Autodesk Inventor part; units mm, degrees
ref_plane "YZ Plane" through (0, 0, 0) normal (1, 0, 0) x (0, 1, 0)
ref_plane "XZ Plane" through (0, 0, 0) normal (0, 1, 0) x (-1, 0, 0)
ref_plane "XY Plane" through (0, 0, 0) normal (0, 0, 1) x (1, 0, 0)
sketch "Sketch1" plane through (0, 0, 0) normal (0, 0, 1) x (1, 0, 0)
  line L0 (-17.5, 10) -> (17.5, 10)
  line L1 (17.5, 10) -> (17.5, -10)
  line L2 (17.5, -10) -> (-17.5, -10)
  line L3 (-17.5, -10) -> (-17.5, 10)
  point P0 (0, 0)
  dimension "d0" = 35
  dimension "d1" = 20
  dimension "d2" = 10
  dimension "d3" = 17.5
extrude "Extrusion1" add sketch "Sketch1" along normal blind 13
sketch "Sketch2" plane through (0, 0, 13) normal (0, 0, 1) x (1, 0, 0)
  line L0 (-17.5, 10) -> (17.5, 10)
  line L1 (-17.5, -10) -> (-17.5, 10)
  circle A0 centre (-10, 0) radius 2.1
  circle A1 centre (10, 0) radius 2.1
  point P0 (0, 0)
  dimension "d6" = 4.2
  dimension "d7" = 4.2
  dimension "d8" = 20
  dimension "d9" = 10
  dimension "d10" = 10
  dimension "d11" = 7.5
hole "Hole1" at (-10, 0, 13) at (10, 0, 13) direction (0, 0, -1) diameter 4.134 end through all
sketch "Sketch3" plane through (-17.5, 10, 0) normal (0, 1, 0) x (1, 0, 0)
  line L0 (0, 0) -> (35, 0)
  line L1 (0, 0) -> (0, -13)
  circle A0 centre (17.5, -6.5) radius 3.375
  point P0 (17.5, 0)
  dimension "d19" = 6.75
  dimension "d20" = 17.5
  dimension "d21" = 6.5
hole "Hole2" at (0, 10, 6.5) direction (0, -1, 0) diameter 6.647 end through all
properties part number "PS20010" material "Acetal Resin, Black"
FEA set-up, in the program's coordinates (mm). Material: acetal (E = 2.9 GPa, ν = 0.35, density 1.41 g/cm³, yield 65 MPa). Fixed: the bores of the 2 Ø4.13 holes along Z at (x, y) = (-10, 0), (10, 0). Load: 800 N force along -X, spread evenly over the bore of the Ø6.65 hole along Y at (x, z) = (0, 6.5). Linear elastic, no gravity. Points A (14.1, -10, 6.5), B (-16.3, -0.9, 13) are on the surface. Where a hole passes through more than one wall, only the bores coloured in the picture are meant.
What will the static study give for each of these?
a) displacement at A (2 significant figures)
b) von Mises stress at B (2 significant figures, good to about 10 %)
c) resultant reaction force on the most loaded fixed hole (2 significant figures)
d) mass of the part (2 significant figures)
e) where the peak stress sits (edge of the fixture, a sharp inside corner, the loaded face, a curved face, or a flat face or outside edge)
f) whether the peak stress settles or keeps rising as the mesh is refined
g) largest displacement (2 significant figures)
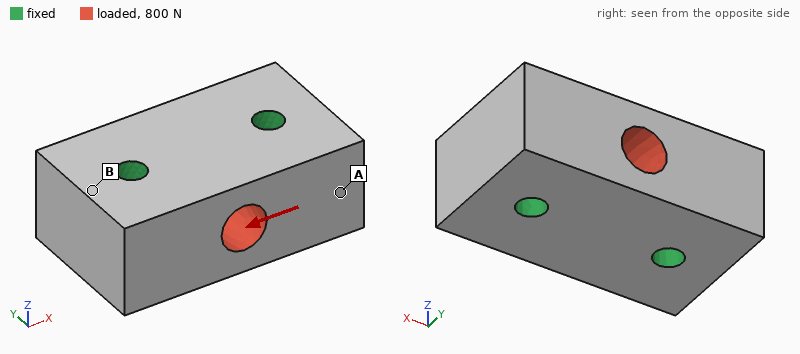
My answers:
5.5 µm
0.98 MPa
400 N
11 g
edge of the fixture
keeps rising
9.6 µm
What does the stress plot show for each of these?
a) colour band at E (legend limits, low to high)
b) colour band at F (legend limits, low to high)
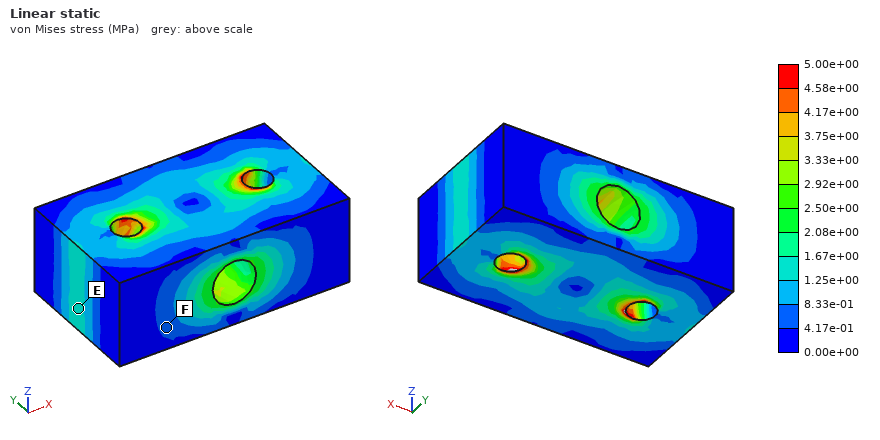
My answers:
1.25e+00 to 1.67e+00 MPa
4.17e-01 to 8.33e-01 MPa
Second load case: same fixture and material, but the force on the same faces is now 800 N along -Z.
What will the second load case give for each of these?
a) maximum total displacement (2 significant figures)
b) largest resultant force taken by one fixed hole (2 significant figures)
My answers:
26 µm
400 N
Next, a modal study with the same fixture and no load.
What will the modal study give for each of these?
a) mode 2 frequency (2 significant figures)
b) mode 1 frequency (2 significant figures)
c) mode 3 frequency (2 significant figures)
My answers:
15 kHz
14 kHz
15 kHz
